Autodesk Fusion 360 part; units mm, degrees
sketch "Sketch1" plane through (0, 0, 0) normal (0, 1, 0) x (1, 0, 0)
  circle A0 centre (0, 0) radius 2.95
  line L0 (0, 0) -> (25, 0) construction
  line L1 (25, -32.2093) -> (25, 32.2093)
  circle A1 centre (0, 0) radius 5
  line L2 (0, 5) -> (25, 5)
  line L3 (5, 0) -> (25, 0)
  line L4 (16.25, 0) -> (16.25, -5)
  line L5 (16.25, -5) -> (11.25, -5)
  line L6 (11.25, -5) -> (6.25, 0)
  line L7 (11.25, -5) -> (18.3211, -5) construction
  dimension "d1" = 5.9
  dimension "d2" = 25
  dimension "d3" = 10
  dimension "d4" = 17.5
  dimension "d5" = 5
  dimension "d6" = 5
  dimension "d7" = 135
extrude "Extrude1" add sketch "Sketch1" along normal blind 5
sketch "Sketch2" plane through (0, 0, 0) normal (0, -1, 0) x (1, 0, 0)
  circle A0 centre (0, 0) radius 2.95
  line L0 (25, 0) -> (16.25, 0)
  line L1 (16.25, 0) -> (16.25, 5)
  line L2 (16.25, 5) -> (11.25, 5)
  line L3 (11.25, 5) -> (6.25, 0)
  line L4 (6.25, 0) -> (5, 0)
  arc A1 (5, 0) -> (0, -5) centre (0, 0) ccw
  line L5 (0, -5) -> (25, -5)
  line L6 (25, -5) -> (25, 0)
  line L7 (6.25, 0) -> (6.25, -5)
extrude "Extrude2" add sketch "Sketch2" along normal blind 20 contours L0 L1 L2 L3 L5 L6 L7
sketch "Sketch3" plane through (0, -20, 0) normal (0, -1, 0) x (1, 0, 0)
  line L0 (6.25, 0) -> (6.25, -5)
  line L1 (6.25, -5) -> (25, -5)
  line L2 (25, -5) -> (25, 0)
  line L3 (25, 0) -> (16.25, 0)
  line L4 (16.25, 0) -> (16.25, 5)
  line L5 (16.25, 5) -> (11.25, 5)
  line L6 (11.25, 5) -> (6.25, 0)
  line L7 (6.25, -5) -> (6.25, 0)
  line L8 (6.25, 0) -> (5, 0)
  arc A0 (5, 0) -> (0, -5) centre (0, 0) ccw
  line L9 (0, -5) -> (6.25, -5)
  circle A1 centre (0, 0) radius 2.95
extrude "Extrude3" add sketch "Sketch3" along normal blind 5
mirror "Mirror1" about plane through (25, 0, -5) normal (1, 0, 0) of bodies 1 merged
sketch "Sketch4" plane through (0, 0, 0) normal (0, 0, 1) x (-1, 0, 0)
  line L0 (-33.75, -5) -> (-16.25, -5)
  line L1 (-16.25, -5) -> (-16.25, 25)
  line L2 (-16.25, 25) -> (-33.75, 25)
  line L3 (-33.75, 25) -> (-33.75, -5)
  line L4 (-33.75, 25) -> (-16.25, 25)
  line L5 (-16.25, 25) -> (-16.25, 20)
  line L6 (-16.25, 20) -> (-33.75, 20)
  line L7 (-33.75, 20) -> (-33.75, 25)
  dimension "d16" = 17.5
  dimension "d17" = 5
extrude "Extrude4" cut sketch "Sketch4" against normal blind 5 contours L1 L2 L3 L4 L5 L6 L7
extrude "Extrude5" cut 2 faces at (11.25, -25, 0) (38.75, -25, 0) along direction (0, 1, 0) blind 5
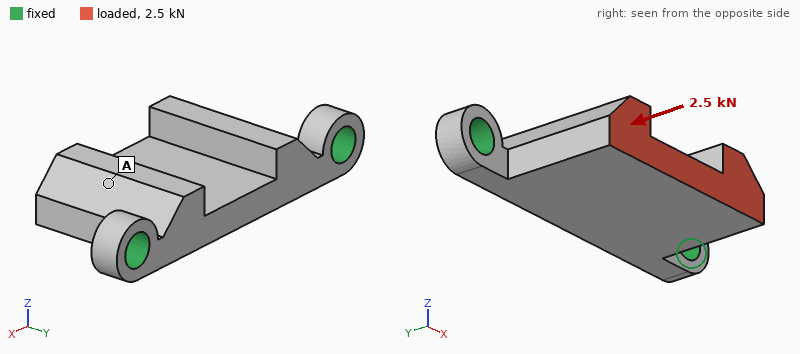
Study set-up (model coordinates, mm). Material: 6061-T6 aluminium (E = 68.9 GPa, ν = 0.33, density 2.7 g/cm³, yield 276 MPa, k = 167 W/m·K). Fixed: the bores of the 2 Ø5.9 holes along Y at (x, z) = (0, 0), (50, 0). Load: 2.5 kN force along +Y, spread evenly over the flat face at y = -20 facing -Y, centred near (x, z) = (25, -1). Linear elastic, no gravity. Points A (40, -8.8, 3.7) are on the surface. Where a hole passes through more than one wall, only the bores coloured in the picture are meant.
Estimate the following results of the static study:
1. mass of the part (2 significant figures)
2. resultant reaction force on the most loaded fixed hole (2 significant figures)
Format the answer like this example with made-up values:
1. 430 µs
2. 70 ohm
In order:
1. 19 g
2. 1.4 kN
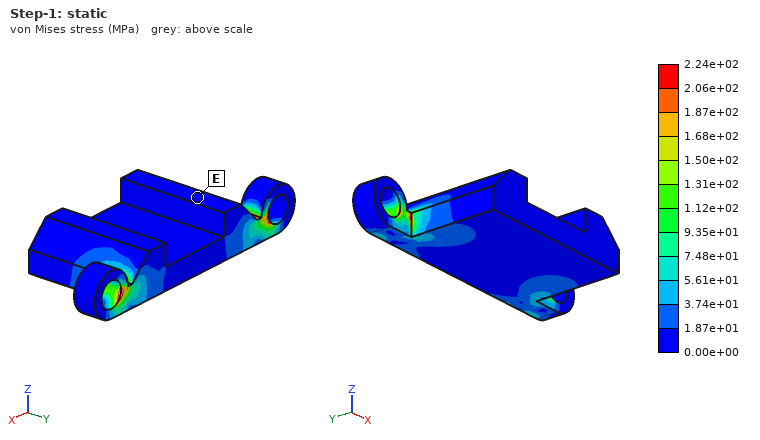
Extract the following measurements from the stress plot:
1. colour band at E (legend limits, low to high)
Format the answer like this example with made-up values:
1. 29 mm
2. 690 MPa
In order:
1. 0.00e+00 to 1.87e+01 MPa
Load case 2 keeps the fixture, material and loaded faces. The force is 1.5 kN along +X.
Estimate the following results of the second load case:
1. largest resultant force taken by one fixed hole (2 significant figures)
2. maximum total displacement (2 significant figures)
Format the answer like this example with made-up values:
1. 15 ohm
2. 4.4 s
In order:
1. 1.1 kN
2. 30 µm
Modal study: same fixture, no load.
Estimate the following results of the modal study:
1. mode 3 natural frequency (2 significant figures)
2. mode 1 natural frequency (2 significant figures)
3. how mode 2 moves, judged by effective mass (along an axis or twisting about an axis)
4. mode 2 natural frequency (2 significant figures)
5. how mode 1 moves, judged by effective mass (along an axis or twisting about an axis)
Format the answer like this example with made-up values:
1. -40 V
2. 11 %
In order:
1. 11 kHz
2. 2800 Hz
3. twisting about Y
4. 9600 Hz
5. along Z
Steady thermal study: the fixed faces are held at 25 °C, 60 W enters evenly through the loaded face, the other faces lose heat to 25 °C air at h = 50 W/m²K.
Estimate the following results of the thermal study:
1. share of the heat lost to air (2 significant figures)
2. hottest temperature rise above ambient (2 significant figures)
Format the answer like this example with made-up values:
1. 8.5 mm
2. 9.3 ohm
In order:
1. 12 %
2. 70 K
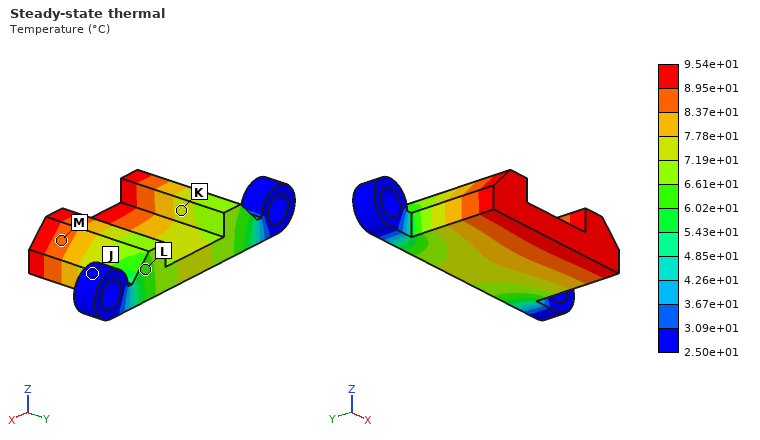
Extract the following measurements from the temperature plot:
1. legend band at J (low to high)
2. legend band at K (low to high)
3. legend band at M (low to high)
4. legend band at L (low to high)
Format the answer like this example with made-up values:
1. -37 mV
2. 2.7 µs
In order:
1. 2.50e+01 to 3.09e+01 °C
2. 7.19e+01 to 7.78e+01 °C
3. 8.37e+01 to 8.95e+01 °C
4. 6.02e+01 to 6.61e+01 °C
